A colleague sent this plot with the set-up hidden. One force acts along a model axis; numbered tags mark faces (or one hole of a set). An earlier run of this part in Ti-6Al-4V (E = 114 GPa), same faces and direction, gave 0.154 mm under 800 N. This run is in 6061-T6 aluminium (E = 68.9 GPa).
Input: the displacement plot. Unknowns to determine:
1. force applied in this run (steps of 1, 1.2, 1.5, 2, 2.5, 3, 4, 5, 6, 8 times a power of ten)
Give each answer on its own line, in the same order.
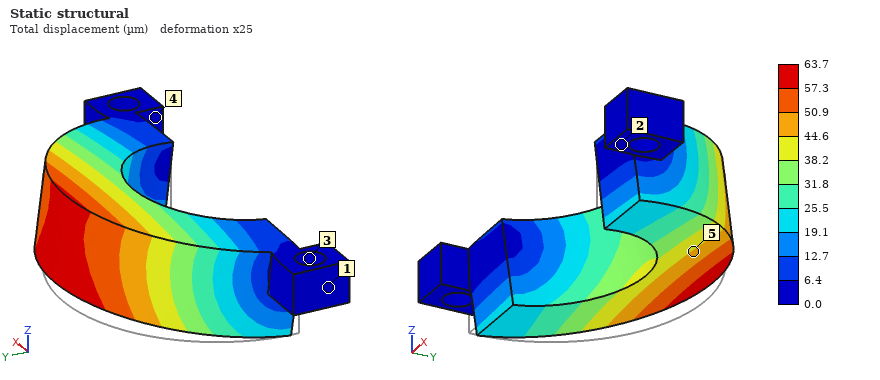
200 N
